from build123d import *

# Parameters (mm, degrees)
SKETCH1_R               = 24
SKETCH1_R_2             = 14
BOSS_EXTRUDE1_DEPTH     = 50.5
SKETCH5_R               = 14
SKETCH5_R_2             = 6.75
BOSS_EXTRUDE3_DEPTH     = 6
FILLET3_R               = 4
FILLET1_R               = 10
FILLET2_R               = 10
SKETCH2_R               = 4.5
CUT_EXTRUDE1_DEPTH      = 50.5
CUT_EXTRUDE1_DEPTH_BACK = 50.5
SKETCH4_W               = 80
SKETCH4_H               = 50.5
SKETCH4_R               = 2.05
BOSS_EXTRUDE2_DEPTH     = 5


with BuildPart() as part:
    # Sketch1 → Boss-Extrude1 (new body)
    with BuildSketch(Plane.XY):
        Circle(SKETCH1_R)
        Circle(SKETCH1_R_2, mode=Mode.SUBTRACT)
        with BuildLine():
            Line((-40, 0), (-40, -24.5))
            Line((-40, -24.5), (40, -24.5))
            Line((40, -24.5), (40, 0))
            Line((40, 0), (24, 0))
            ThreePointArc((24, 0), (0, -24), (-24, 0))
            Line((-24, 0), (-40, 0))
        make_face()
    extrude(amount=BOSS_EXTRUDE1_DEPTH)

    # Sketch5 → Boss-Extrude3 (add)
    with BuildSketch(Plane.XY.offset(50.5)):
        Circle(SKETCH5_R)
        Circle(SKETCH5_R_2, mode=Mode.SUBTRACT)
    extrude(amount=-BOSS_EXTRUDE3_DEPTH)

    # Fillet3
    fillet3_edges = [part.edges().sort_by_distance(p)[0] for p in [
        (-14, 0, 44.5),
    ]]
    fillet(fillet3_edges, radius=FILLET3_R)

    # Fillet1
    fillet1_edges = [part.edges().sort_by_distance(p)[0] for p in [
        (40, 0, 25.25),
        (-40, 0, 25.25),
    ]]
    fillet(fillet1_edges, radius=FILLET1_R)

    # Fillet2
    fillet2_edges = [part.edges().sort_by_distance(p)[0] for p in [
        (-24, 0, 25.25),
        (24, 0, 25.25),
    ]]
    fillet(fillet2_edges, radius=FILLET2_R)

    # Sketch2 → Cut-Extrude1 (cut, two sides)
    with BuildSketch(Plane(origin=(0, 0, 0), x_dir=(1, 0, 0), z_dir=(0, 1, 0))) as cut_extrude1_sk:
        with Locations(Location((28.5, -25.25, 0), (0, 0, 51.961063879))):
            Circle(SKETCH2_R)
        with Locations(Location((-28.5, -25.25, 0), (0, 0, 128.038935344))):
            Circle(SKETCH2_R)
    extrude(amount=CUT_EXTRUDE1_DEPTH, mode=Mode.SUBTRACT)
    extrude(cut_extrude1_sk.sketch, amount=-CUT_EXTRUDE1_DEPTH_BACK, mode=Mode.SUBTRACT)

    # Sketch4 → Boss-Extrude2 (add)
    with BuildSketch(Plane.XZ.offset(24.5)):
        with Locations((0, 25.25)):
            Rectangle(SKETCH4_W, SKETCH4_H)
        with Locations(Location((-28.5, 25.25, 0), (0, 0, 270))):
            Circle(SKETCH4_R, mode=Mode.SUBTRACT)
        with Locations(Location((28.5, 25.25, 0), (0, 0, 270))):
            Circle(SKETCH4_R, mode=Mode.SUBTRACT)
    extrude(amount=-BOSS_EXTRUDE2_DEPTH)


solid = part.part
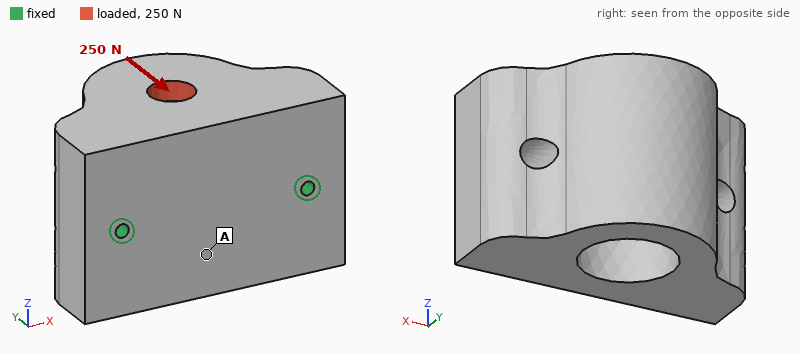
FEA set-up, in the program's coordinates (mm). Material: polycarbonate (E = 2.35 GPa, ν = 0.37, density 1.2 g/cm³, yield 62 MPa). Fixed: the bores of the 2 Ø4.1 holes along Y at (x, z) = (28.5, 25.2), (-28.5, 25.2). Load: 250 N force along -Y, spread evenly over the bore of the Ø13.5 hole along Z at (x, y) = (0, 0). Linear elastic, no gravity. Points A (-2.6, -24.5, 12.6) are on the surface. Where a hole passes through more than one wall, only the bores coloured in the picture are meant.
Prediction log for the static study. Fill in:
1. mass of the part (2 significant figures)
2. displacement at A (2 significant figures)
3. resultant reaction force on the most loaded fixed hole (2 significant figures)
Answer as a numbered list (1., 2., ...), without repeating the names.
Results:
1. 140 g
2. 0.15 mm
3. 130 N
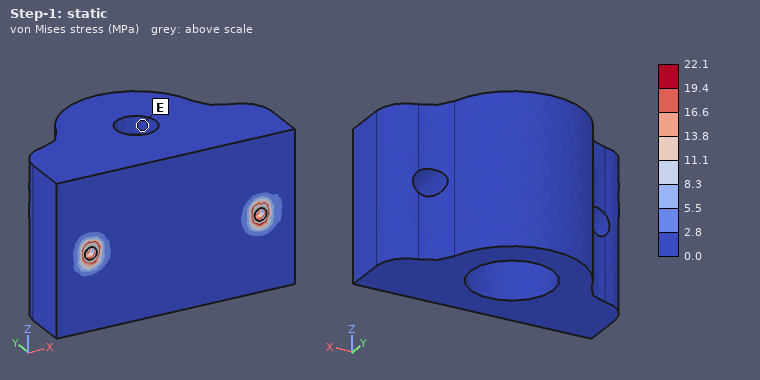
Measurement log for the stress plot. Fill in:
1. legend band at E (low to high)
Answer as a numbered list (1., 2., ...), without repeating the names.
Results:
1. 0.0 to 2.8 MPa
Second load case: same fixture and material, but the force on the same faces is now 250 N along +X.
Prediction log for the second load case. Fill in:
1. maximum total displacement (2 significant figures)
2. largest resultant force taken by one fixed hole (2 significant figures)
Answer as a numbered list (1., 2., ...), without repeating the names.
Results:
1. 31 µm
2. 180 N
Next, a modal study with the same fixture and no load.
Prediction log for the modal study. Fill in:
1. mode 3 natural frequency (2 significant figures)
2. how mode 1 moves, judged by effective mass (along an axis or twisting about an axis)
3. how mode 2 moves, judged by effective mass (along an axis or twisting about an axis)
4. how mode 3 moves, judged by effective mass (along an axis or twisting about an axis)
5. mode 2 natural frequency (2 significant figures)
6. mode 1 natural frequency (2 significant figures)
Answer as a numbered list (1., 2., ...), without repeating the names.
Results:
1. 2100 Hz
2. along Z
3. along X
4. along Y
5. 1800 Hz
6. 350 Hz
